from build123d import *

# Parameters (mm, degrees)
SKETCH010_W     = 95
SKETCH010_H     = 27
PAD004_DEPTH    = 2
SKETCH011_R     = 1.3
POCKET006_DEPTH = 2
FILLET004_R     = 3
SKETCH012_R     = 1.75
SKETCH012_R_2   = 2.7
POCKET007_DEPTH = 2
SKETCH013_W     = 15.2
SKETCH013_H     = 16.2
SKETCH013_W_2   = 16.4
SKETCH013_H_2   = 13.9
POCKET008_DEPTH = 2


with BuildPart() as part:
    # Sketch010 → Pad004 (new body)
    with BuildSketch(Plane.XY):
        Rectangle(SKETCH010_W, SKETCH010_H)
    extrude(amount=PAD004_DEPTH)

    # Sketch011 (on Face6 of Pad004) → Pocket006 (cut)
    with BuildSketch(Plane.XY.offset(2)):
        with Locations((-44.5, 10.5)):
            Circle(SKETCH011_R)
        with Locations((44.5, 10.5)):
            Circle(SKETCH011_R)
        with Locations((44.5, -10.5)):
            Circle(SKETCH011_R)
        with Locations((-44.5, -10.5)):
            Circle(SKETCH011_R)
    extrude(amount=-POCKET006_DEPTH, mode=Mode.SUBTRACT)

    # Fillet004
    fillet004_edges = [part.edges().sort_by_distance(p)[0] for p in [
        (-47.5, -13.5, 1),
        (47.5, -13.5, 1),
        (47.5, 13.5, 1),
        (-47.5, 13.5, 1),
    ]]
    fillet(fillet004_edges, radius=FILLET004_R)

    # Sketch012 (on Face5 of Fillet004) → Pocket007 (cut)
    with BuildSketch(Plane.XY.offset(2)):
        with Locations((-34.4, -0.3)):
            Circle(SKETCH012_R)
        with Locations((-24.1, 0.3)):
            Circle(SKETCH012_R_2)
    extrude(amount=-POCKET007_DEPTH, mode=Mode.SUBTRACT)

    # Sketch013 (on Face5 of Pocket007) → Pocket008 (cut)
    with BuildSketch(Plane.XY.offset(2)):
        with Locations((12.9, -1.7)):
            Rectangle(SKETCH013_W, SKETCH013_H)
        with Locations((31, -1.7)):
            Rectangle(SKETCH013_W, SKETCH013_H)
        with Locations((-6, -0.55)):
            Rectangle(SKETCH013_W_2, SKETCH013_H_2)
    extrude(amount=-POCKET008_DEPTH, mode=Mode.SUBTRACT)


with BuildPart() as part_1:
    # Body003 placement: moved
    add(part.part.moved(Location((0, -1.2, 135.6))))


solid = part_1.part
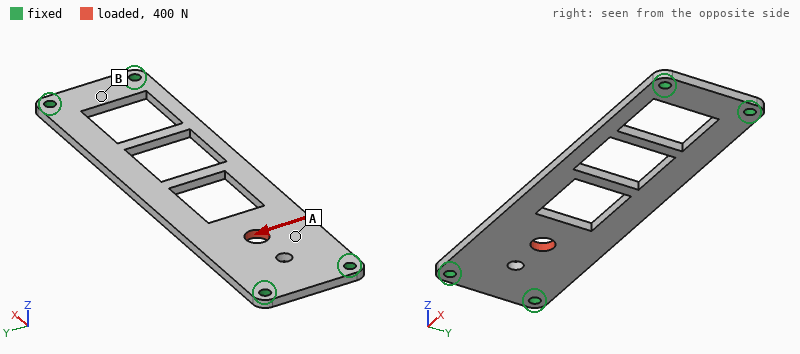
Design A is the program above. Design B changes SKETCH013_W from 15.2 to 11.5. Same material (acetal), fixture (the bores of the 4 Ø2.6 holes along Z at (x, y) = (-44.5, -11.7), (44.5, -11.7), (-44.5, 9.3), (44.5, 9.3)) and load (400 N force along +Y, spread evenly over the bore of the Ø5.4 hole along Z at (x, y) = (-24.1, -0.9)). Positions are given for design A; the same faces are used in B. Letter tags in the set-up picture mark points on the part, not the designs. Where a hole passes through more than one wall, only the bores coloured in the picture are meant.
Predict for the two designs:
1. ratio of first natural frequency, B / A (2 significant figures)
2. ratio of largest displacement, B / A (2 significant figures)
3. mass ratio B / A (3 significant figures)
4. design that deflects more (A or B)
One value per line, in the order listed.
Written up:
0.98
0.90
1.07
A
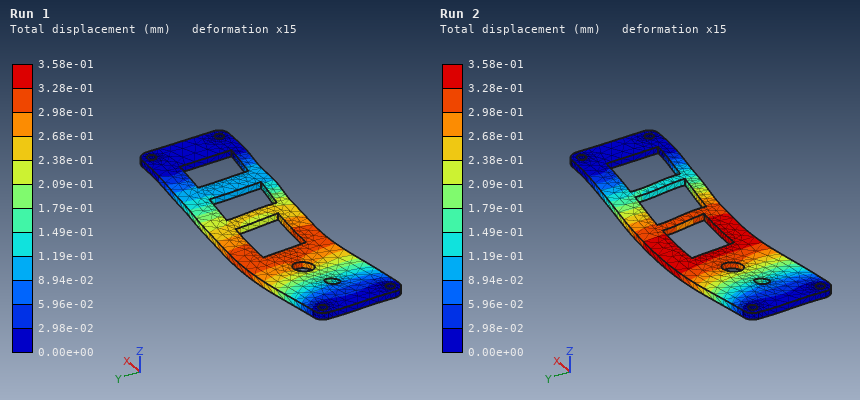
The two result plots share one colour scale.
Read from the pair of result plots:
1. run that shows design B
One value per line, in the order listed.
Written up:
Run 1
